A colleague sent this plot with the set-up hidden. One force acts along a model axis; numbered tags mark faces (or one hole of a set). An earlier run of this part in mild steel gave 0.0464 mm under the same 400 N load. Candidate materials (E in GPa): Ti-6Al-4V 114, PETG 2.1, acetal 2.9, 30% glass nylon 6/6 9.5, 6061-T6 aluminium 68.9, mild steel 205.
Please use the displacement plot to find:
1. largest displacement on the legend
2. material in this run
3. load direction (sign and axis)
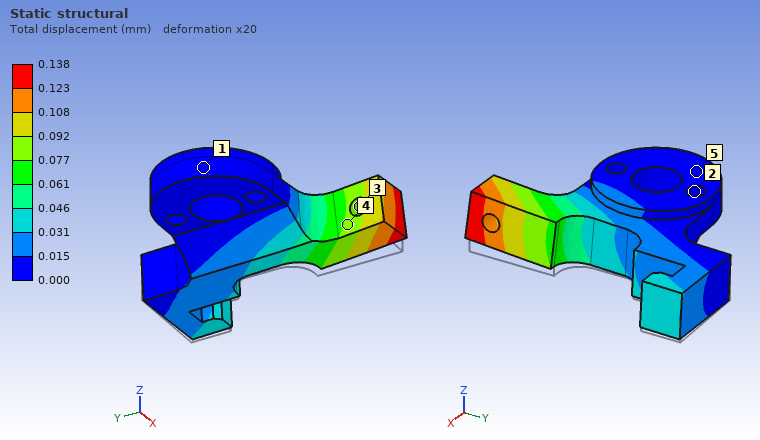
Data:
0.138 mm
6061-T6 aluminium
+Z
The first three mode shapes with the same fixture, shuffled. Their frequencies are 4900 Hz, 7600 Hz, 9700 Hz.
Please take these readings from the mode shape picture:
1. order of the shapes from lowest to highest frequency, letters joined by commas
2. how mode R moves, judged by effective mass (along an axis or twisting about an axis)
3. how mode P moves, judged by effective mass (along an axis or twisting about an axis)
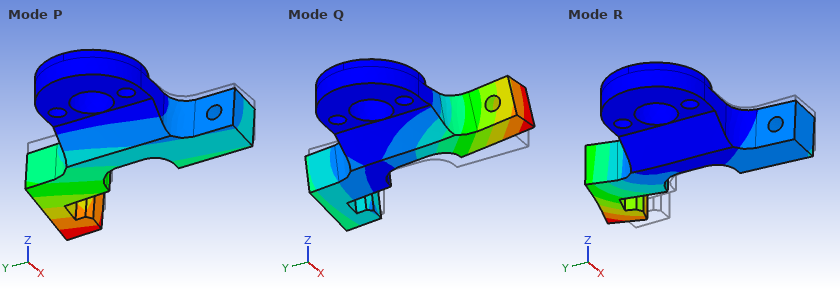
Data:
P, Q, R
along Y
along Z
